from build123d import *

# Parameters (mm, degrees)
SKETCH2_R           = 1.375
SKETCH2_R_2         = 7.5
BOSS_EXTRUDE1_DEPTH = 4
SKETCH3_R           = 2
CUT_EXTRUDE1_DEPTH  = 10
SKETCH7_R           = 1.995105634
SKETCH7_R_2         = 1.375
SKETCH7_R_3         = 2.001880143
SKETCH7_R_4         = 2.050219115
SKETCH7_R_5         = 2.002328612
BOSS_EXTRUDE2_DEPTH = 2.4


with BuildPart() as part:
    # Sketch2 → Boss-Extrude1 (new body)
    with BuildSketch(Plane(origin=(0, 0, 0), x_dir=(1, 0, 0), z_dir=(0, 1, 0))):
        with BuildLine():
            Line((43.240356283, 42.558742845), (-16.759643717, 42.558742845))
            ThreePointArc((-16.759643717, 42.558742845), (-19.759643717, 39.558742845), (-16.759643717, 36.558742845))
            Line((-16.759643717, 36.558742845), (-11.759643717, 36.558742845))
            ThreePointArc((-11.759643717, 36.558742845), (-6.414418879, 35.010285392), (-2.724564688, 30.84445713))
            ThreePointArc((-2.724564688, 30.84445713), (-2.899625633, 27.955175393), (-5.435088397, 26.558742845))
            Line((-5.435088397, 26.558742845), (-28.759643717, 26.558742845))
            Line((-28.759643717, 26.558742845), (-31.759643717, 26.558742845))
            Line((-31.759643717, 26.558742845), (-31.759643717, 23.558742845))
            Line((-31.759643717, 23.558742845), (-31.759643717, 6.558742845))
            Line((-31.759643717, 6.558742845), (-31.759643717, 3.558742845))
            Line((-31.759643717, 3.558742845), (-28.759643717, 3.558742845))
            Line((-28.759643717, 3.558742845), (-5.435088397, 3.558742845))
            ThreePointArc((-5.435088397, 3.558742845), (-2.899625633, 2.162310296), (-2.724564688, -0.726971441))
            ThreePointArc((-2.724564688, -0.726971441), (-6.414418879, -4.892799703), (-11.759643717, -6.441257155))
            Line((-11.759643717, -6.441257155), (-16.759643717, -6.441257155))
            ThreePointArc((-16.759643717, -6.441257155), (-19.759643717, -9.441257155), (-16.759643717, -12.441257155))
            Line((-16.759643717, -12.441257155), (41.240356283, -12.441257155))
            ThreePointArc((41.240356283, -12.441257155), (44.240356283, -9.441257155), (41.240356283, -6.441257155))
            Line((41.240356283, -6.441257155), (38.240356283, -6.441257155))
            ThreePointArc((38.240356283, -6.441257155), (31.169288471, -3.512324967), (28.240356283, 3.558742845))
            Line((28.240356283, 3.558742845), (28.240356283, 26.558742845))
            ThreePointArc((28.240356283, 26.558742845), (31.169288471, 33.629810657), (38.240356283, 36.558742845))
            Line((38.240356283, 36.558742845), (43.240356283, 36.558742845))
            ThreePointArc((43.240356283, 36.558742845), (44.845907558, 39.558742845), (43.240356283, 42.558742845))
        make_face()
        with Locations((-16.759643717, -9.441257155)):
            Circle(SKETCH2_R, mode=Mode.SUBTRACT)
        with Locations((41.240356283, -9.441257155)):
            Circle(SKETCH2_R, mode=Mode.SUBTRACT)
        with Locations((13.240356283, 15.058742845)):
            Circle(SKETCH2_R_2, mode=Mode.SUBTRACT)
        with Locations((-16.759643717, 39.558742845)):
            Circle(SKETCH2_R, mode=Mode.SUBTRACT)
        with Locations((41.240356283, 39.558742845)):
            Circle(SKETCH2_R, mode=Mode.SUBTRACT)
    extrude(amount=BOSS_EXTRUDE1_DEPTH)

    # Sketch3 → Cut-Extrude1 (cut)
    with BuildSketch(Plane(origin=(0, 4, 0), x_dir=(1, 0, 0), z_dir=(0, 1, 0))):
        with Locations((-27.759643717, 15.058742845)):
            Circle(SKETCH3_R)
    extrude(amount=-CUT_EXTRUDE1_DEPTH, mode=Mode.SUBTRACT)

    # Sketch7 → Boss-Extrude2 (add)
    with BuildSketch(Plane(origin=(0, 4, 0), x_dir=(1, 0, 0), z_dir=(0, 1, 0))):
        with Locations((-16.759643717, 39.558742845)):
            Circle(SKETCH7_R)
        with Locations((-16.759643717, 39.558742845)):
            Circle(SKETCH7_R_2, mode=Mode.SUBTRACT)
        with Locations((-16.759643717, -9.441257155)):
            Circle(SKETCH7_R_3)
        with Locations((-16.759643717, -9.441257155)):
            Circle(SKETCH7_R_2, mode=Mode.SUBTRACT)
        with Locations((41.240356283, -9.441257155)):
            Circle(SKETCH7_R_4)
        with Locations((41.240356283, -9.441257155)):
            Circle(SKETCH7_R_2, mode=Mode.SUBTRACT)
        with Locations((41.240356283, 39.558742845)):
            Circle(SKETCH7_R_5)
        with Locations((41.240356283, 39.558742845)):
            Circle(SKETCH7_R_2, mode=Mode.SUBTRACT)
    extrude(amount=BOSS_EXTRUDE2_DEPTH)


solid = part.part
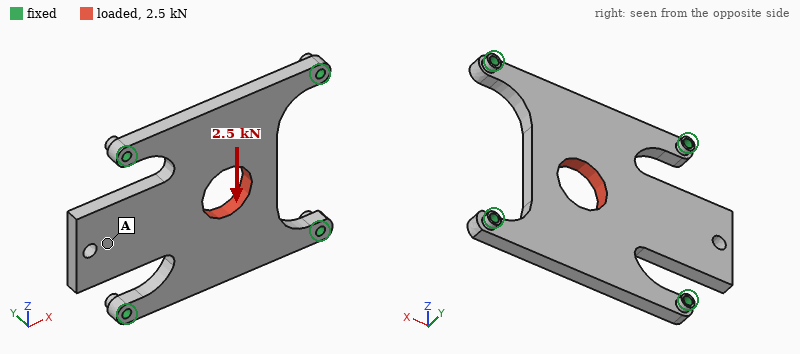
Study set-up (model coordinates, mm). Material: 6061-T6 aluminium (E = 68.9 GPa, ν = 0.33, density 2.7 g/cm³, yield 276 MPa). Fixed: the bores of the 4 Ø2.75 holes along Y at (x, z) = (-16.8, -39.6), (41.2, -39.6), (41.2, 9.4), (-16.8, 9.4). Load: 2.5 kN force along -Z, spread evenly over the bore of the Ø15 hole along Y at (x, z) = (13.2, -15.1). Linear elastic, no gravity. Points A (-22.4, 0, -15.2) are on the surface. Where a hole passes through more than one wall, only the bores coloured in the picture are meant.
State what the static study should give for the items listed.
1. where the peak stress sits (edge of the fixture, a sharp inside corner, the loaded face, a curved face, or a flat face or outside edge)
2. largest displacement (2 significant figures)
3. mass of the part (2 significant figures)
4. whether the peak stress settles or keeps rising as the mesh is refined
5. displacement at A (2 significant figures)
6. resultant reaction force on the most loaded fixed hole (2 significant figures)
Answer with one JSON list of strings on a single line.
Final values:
["edge of the fixture", "41 µm", "28 g", "keeps rising", "39 µm", "910 N"]
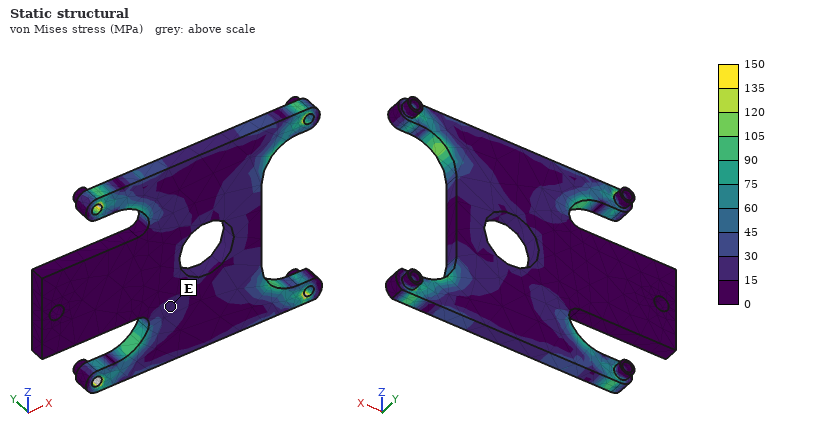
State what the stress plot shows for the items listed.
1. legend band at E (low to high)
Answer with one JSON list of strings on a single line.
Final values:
["15 to 30 MPa"]
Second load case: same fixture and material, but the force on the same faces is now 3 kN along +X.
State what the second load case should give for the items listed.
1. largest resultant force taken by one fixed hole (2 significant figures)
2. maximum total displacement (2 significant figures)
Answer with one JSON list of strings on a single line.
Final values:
["830 N", "21 µm"]
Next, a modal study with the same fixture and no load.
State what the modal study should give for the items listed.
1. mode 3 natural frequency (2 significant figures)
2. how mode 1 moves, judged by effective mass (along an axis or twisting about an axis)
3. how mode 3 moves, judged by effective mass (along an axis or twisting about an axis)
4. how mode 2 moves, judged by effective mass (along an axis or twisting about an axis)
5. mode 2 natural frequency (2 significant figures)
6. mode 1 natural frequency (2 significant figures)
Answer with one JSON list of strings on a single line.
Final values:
["5700 Hz", "along Y", "twisting about X", "along Y", "3600 Hz", "1800 Hz"]
